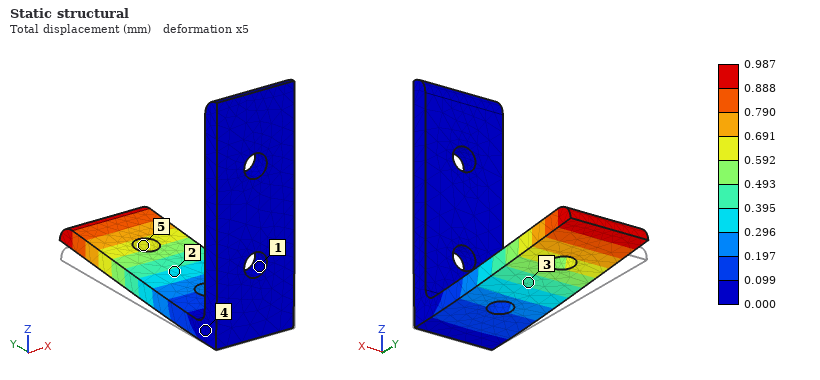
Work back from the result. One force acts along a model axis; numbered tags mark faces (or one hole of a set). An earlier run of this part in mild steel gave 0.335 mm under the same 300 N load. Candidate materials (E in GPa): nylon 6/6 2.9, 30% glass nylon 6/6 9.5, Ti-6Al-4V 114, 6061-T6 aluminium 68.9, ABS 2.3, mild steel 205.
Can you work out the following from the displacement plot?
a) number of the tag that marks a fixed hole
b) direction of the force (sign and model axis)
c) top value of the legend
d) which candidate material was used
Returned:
1
+Z
0.987 mm
6061-T6 aluminium
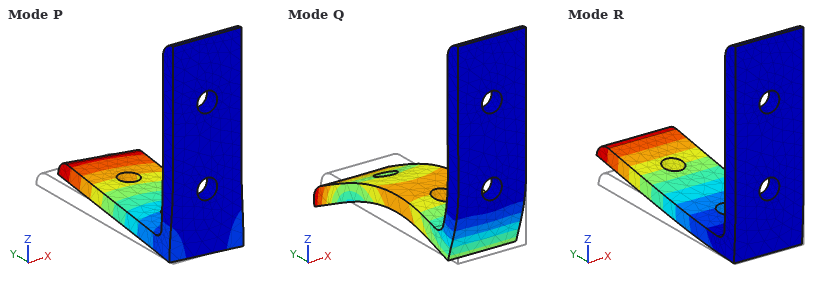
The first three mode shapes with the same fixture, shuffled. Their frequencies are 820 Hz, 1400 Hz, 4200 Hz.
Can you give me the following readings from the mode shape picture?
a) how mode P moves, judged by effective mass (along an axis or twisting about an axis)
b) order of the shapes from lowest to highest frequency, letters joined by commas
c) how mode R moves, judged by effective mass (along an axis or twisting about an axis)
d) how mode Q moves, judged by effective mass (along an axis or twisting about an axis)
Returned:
along X
R, P, Q
along Z
along Y
